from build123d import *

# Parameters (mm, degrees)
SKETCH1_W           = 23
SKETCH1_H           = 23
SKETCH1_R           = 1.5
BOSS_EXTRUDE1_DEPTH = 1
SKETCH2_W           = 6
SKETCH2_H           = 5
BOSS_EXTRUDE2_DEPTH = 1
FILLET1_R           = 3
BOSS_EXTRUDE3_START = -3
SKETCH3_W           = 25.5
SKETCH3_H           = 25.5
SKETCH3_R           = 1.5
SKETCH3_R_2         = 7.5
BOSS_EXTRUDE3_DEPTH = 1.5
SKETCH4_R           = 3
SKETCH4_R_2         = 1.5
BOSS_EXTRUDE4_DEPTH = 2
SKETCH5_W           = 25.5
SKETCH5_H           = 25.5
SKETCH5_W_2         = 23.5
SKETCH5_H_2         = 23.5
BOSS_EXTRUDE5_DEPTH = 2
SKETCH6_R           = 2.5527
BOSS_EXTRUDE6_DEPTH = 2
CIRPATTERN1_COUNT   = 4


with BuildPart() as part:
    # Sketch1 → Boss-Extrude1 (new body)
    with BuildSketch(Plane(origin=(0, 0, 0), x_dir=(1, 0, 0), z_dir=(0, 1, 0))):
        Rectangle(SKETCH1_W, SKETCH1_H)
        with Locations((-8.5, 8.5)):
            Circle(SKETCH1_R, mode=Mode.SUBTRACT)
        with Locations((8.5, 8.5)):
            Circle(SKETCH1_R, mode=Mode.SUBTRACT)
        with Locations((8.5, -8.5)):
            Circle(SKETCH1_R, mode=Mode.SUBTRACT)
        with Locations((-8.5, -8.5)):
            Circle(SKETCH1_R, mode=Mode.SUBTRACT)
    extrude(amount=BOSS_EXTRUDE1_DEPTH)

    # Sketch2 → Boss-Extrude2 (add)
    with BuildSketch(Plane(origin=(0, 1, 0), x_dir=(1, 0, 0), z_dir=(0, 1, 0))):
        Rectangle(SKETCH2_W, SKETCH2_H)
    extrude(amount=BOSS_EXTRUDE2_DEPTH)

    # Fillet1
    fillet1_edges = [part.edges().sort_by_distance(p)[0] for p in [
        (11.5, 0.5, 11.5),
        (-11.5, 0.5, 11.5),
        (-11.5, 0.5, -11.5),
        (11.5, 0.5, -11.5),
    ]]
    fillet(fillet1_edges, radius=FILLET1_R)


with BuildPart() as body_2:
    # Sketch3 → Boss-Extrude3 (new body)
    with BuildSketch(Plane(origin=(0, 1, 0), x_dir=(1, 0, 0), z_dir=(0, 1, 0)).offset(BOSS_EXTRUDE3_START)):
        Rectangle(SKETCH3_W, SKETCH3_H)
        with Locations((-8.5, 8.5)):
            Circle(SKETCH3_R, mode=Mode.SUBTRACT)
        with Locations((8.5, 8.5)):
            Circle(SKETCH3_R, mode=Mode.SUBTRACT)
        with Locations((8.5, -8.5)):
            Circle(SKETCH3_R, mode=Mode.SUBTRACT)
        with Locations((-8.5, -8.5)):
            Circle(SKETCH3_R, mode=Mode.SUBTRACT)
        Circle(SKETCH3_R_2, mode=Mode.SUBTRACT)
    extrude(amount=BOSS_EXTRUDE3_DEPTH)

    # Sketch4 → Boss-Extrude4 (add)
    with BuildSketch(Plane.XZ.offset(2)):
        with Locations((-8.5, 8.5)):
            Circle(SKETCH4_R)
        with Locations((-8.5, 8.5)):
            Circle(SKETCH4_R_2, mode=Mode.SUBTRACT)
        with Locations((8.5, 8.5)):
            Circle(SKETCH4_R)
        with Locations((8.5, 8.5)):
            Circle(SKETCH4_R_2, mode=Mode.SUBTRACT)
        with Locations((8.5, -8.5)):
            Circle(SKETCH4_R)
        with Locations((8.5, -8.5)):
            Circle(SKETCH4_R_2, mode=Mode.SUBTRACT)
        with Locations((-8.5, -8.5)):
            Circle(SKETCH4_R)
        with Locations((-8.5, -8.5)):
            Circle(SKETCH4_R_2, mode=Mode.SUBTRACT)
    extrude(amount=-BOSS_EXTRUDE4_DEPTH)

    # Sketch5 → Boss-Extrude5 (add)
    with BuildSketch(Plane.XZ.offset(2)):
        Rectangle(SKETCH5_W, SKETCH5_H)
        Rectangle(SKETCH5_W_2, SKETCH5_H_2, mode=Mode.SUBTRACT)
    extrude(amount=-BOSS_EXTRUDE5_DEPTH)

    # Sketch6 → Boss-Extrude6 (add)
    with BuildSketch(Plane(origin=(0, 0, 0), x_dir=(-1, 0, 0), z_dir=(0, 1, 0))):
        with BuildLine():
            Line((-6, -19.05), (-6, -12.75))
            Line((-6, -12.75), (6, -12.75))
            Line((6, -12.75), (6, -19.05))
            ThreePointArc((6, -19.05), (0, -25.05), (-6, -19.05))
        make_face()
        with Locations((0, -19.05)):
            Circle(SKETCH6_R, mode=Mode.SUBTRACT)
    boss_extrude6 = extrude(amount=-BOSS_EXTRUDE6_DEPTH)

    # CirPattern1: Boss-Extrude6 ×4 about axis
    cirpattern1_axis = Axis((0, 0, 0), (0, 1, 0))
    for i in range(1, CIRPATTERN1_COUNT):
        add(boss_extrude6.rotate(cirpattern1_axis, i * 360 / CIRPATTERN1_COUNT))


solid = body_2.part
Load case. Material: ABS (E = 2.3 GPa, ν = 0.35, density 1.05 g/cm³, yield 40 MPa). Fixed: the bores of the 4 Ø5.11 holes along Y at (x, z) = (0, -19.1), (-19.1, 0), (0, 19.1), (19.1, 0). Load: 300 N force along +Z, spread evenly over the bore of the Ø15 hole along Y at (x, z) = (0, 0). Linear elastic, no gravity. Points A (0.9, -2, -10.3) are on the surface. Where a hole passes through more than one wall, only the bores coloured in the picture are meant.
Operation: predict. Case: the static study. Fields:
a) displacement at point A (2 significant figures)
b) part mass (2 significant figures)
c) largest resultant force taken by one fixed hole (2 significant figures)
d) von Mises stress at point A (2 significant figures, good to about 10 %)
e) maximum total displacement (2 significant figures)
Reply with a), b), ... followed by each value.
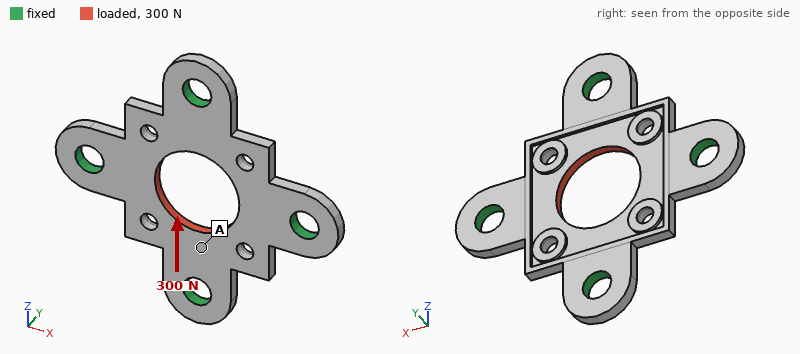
a) 22 µm
b) 1.7 g
c) 110 N
d) 5.3 MPa
e) 47 µm
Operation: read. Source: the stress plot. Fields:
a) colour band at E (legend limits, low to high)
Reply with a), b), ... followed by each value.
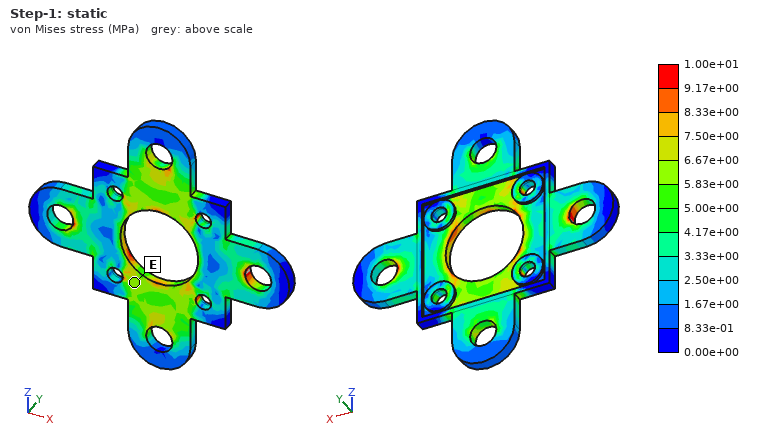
a) 5.83e+00 to 6.67e+00 MPa
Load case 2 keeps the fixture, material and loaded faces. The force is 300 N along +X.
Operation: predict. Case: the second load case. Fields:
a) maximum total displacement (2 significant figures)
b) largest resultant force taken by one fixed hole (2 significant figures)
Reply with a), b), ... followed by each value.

a) 47 µm
b) 110 N
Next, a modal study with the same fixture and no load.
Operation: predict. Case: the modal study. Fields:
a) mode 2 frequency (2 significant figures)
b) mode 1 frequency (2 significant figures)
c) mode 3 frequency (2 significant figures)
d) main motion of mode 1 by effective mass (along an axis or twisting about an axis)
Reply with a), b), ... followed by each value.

a) 5400 Hz
b) 4800 Hz
c) 5400 Hz
d) along Y
